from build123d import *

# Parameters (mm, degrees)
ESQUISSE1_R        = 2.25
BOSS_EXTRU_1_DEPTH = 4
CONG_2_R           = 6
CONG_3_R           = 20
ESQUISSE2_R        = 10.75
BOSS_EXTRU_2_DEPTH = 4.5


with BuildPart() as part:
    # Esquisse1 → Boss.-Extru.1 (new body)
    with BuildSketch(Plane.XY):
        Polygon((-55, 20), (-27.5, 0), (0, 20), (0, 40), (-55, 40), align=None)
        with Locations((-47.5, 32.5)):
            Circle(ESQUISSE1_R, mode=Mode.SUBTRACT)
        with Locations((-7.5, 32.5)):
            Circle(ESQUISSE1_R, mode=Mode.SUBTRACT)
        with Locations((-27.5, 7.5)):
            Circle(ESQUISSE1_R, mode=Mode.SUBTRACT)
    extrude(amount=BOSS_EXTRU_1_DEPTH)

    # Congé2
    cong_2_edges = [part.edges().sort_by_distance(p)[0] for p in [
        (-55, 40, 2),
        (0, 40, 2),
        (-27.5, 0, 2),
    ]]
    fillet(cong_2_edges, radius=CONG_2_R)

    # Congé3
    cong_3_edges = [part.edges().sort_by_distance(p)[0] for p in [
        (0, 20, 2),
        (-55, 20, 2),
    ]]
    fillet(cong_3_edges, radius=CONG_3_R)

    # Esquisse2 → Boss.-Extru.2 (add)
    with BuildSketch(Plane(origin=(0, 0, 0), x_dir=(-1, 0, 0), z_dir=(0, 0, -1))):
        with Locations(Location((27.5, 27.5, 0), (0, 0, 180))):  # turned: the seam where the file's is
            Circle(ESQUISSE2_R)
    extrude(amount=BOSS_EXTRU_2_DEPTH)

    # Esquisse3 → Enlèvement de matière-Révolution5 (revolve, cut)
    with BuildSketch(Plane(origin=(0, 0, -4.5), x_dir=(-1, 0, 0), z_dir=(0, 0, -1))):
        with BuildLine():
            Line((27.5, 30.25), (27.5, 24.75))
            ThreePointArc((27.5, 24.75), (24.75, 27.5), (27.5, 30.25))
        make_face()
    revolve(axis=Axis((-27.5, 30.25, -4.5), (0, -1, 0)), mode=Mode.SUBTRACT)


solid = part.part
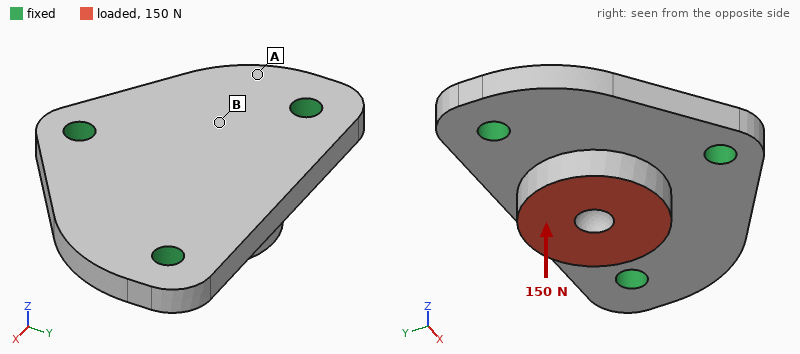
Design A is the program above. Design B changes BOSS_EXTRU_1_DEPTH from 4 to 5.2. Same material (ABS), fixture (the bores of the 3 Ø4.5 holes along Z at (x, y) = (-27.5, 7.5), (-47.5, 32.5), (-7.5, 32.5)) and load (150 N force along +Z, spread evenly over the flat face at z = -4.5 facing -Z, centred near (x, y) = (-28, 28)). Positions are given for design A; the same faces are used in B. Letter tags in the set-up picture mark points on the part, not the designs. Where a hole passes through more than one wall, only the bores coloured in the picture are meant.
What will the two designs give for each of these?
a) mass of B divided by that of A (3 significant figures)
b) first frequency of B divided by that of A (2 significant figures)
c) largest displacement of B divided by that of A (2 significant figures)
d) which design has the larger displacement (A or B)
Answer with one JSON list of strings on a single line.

["1.24", "1.2", "0.59", "A"]
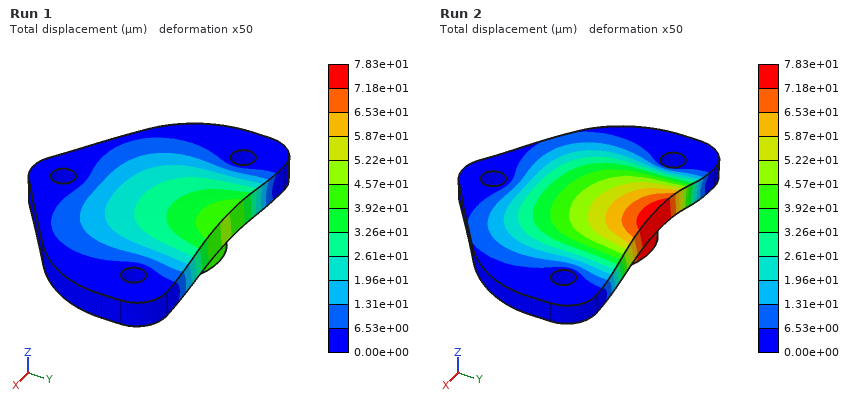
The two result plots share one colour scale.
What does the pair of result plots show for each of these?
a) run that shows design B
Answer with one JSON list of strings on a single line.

["Run 1"]
